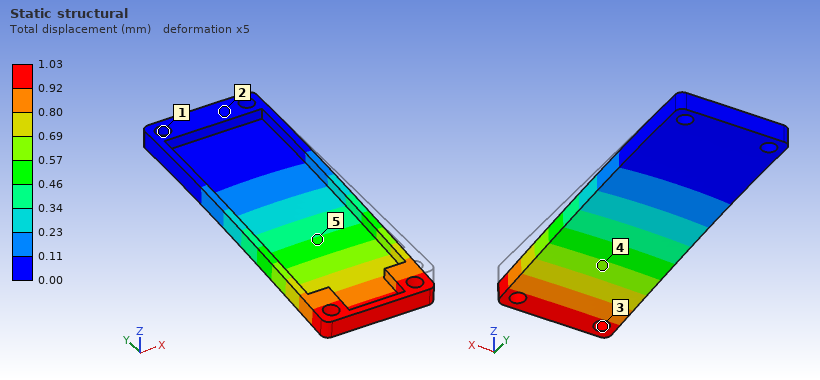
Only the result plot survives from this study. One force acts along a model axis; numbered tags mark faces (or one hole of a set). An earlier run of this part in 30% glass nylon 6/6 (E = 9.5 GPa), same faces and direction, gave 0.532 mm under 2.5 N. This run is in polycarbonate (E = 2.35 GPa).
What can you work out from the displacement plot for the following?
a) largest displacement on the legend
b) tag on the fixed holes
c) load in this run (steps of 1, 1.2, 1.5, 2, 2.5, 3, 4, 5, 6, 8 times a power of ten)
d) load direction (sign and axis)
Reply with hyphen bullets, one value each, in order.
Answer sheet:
- 1.03 mm
- 1
- 1.2 N
- -Z
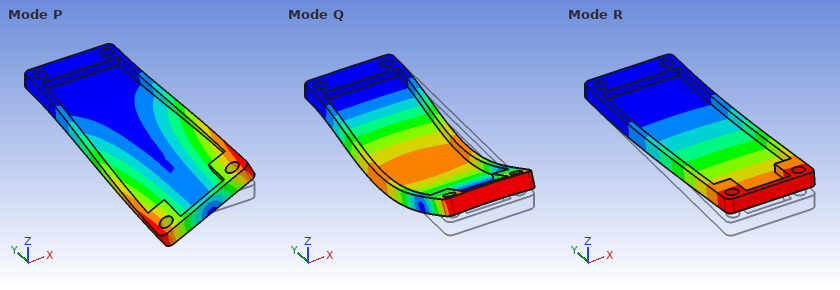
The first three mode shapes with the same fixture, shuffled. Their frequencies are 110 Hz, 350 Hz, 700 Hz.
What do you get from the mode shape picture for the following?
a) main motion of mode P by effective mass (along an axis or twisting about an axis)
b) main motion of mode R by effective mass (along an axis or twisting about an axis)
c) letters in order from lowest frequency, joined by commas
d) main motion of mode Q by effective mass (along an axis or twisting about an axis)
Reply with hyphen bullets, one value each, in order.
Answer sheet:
- twisting about Y
- along Z
- R, P, Q
- along Z
